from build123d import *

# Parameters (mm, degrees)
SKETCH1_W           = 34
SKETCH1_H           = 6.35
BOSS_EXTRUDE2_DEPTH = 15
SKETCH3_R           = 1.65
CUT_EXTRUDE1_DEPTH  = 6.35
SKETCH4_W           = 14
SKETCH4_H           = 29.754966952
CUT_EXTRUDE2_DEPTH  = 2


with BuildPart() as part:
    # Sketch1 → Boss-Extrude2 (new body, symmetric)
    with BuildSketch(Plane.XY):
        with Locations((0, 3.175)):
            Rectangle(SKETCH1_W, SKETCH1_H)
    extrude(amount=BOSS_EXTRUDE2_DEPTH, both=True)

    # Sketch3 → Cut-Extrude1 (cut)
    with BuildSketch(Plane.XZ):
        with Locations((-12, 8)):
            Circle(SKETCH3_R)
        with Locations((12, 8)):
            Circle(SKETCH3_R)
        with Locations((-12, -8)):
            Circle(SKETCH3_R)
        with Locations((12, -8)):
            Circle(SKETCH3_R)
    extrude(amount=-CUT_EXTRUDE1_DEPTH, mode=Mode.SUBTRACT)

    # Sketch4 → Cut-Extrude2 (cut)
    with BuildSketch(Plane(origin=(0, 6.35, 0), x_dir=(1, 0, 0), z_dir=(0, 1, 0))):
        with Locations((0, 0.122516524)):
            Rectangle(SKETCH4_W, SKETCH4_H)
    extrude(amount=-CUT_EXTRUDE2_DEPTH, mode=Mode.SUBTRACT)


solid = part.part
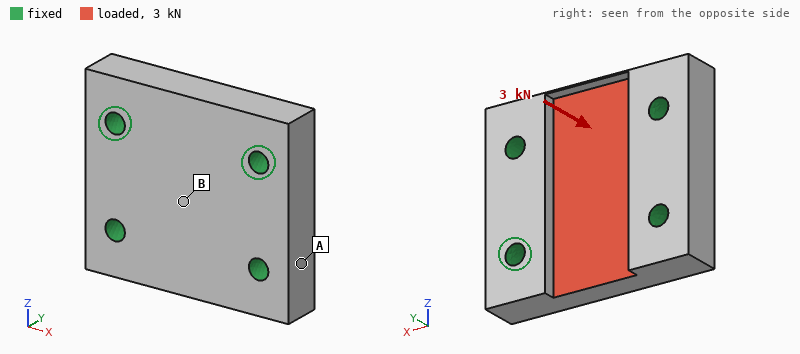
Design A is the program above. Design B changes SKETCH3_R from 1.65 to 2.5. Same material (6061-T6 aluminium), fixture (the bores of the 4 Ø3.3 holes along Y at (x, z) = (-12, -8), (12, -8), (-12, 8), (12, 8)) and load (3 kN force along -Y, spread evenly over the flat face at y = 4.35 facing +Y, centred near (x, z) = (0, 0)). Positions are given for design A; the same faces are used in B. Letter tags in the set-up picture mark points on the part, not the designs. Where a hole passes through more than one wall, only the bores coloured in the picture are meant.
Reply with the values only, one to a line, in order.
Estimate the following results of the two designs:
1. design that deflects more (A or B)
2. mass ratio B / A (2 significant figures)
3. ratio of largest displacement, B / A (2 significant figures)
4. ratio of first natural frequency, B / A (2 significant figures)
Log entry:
A
0.95
0.78
1.2
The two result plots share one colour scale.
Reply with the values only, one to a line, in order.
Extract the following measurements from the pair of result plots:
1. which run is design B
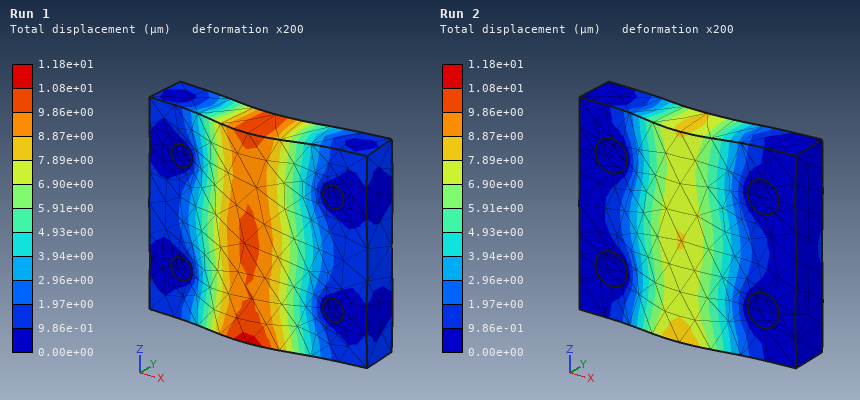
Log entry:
Run 2
